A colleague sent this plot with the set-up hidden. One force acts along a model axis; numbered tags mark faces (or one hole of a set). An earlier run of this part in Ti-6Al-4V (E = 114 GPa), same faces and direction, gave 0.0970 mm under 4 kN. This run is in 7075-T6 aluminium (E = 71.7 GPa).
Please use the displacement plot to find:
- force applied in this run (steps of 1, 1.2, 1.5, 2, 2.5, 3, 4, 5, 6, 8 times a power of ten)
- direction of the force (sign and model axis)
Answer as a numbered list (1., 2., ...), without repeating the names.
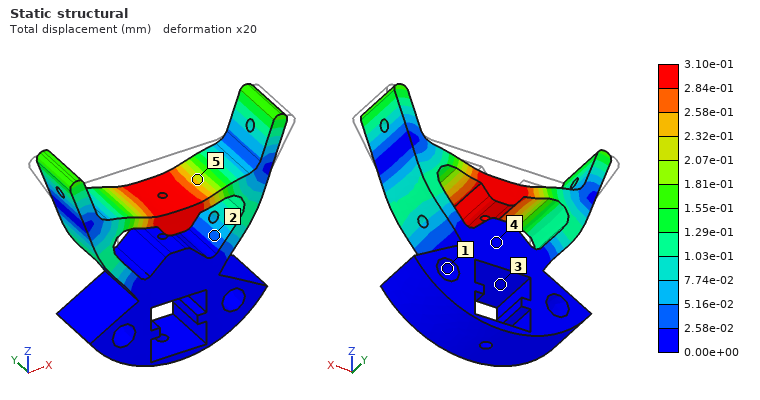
1. 8 kN
2. -Z
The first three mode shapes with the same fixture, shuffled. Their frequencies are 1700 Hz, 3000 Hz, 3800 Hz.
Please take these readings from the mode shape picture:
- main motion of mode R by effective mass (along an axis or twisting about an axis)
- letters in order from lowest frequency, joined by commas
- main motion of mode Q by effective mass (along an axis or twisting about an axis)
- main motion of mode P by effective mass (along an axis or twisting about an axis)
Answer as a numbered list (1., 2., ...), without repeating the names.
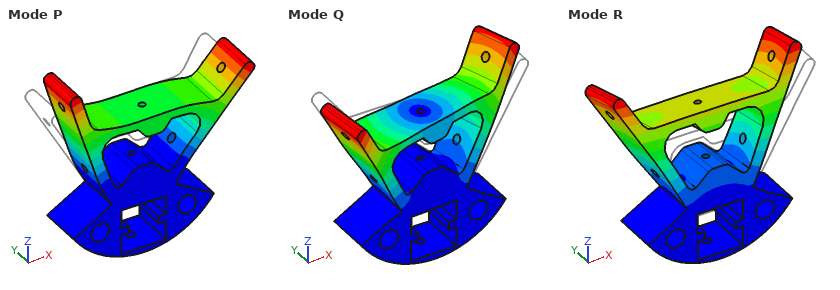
1. along Y
2. P, R, Q
3. twisting about Z
4. along X
